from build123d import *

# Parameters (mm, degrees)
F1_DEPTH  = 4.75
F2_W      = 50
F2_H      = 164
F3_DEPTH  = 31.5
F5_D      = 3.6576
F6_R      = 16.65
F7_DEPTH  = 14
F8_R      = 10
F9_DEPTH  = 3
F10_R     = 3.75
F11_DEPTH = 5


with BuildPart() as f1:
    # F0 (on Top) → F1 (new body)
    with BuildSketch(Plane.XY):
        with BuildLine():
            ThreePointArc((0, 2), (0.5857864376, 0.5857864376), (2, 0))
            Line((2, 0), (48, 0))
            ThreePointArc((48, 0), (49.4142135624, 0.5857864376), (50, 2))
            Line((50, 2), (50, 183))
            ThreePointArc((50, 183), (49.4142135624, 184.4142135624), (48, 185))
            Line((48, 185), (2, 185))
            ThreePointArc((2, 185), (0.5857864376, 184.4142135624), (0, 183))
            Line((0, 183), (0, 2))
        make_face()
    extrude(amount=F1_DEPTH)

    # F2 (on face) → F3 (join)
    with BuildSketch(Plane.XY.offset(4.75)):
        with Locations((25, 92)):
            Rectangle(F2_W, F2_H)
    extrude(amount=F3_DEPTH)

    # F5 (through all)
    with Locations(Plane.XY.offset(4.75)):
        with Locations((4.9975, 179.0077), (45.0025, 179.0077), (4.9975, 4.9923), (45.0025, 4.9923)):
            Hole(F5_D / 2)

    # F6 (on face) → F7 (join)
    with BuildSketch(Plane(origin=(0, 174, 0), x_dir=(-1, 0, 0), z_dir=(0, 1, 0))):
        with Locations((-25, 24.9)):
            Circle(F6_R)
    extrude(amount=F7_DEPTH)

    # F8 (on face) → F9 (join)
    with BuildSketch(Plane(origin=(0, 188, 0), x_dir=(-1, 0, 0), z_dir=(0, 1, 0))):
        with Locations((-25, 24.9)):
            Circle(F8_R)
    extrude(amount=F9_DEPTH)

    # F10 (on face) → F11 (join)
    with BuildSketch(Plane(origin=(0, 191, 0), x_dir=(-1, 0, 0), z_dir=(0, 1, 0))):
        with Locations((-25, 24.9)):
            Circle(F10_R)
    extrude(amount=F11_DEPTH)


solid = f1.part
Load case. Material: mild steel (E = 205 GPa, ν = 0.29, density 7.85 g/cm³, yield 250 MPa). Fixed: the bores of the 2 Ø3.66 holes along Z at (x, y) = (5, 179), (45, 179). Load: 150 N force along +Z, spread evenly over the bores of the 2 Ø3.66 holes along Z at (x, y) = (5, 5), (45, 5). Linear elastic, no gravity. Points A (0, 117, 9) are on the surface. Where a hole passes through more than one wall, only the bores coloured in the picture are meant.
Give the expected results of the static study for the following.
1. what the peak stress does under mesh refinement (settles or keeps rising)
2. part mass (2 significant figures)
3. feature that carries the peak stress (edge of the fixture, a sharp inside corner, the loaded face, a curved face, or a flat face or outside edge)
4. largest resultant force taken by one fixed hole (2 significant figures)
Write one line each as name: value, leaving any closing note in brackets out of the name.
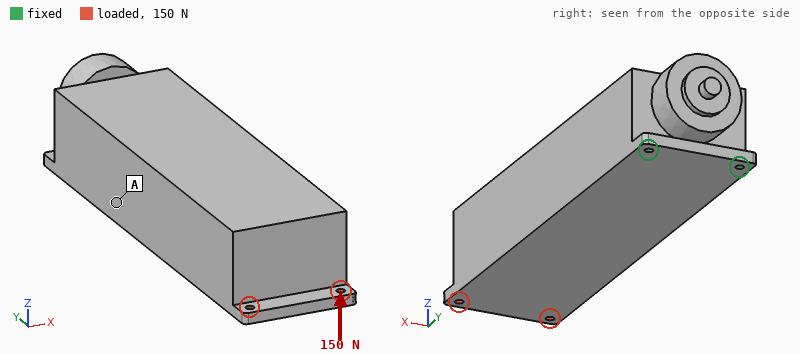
what the peak stress does under mesh refinement: keeps rising
part mass: 2.5 kg
feature that carries the peak stress: edge of the fixture
largest resultant force taken by one fixed hole: 80 N
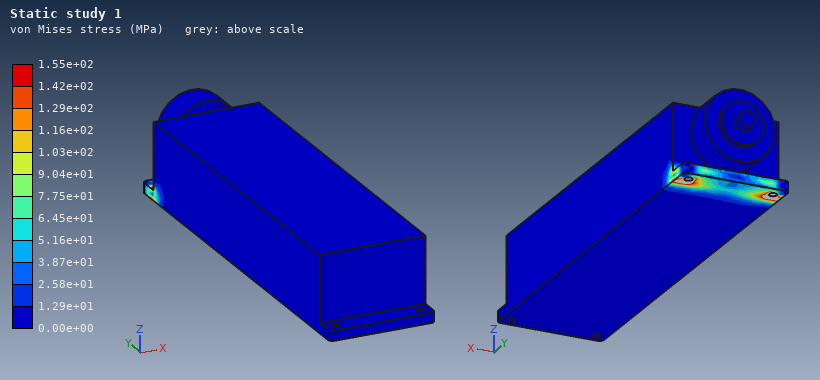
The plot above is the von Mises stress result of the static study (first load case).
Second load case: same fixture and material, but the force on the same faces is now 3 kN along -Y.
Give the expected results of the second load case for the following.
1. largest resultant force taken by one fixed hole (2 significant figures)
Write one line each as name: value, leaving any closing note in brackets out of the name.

largest resultant force taken by one fixed hole: 1.5 kN
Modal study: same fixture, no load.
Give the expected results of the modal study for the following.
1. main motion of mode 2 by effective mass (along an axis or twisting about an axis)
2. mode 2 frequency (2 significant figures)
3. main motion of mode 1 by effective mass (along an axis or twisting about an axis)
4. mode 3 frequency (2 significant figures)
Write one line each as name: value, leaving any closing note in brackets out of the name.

main motion of mode 2 by effective mass: along X
mode 2 frequency: 740 Hz
main motion of mode 1 by effective mass: along Z
mode 3 frequency: 2100 Hz
